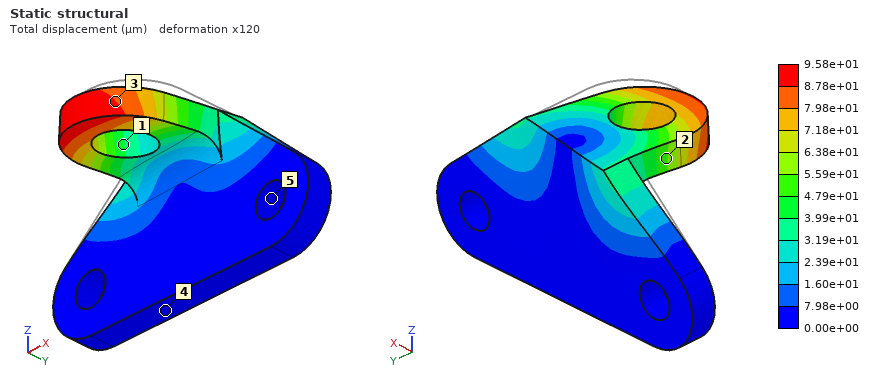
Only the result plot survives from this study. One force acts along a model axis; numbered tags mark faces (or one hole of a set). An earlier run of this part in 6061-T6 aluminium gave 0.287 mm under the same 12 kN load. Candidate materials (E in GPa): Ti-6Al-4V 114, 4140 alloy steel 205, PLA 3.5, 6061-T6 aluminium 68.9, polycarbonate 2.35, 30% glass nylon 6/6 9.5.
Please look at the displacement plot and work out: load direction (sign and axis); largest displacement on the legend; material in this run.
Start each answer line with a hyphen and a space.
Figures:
- -X
- 9.58e+01 µm
- 4140 alloy steel
